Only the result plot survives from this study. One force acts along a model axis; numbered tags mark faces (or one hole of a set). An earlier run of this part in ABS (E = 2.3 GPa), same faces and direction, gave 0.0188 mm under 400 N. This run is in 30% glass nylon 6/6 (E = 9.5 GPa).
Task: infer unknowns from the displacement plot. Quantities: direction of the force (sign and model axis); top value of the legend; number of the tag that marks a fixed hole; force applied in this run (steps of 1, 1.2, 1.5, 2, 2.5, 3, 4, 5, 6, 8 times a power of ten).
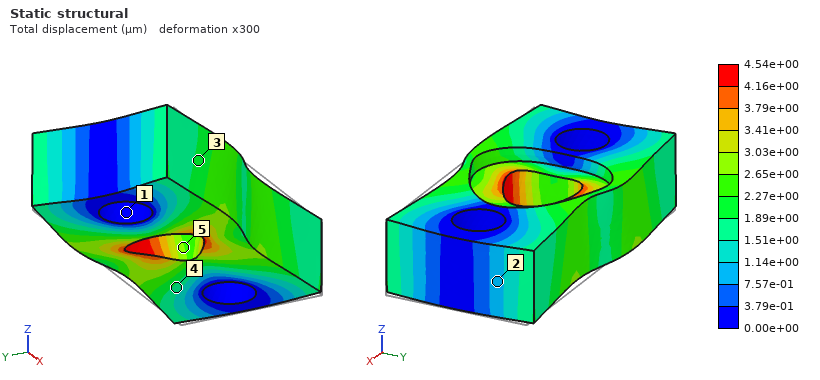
-X
4.54e+00 µm
1
400 N
